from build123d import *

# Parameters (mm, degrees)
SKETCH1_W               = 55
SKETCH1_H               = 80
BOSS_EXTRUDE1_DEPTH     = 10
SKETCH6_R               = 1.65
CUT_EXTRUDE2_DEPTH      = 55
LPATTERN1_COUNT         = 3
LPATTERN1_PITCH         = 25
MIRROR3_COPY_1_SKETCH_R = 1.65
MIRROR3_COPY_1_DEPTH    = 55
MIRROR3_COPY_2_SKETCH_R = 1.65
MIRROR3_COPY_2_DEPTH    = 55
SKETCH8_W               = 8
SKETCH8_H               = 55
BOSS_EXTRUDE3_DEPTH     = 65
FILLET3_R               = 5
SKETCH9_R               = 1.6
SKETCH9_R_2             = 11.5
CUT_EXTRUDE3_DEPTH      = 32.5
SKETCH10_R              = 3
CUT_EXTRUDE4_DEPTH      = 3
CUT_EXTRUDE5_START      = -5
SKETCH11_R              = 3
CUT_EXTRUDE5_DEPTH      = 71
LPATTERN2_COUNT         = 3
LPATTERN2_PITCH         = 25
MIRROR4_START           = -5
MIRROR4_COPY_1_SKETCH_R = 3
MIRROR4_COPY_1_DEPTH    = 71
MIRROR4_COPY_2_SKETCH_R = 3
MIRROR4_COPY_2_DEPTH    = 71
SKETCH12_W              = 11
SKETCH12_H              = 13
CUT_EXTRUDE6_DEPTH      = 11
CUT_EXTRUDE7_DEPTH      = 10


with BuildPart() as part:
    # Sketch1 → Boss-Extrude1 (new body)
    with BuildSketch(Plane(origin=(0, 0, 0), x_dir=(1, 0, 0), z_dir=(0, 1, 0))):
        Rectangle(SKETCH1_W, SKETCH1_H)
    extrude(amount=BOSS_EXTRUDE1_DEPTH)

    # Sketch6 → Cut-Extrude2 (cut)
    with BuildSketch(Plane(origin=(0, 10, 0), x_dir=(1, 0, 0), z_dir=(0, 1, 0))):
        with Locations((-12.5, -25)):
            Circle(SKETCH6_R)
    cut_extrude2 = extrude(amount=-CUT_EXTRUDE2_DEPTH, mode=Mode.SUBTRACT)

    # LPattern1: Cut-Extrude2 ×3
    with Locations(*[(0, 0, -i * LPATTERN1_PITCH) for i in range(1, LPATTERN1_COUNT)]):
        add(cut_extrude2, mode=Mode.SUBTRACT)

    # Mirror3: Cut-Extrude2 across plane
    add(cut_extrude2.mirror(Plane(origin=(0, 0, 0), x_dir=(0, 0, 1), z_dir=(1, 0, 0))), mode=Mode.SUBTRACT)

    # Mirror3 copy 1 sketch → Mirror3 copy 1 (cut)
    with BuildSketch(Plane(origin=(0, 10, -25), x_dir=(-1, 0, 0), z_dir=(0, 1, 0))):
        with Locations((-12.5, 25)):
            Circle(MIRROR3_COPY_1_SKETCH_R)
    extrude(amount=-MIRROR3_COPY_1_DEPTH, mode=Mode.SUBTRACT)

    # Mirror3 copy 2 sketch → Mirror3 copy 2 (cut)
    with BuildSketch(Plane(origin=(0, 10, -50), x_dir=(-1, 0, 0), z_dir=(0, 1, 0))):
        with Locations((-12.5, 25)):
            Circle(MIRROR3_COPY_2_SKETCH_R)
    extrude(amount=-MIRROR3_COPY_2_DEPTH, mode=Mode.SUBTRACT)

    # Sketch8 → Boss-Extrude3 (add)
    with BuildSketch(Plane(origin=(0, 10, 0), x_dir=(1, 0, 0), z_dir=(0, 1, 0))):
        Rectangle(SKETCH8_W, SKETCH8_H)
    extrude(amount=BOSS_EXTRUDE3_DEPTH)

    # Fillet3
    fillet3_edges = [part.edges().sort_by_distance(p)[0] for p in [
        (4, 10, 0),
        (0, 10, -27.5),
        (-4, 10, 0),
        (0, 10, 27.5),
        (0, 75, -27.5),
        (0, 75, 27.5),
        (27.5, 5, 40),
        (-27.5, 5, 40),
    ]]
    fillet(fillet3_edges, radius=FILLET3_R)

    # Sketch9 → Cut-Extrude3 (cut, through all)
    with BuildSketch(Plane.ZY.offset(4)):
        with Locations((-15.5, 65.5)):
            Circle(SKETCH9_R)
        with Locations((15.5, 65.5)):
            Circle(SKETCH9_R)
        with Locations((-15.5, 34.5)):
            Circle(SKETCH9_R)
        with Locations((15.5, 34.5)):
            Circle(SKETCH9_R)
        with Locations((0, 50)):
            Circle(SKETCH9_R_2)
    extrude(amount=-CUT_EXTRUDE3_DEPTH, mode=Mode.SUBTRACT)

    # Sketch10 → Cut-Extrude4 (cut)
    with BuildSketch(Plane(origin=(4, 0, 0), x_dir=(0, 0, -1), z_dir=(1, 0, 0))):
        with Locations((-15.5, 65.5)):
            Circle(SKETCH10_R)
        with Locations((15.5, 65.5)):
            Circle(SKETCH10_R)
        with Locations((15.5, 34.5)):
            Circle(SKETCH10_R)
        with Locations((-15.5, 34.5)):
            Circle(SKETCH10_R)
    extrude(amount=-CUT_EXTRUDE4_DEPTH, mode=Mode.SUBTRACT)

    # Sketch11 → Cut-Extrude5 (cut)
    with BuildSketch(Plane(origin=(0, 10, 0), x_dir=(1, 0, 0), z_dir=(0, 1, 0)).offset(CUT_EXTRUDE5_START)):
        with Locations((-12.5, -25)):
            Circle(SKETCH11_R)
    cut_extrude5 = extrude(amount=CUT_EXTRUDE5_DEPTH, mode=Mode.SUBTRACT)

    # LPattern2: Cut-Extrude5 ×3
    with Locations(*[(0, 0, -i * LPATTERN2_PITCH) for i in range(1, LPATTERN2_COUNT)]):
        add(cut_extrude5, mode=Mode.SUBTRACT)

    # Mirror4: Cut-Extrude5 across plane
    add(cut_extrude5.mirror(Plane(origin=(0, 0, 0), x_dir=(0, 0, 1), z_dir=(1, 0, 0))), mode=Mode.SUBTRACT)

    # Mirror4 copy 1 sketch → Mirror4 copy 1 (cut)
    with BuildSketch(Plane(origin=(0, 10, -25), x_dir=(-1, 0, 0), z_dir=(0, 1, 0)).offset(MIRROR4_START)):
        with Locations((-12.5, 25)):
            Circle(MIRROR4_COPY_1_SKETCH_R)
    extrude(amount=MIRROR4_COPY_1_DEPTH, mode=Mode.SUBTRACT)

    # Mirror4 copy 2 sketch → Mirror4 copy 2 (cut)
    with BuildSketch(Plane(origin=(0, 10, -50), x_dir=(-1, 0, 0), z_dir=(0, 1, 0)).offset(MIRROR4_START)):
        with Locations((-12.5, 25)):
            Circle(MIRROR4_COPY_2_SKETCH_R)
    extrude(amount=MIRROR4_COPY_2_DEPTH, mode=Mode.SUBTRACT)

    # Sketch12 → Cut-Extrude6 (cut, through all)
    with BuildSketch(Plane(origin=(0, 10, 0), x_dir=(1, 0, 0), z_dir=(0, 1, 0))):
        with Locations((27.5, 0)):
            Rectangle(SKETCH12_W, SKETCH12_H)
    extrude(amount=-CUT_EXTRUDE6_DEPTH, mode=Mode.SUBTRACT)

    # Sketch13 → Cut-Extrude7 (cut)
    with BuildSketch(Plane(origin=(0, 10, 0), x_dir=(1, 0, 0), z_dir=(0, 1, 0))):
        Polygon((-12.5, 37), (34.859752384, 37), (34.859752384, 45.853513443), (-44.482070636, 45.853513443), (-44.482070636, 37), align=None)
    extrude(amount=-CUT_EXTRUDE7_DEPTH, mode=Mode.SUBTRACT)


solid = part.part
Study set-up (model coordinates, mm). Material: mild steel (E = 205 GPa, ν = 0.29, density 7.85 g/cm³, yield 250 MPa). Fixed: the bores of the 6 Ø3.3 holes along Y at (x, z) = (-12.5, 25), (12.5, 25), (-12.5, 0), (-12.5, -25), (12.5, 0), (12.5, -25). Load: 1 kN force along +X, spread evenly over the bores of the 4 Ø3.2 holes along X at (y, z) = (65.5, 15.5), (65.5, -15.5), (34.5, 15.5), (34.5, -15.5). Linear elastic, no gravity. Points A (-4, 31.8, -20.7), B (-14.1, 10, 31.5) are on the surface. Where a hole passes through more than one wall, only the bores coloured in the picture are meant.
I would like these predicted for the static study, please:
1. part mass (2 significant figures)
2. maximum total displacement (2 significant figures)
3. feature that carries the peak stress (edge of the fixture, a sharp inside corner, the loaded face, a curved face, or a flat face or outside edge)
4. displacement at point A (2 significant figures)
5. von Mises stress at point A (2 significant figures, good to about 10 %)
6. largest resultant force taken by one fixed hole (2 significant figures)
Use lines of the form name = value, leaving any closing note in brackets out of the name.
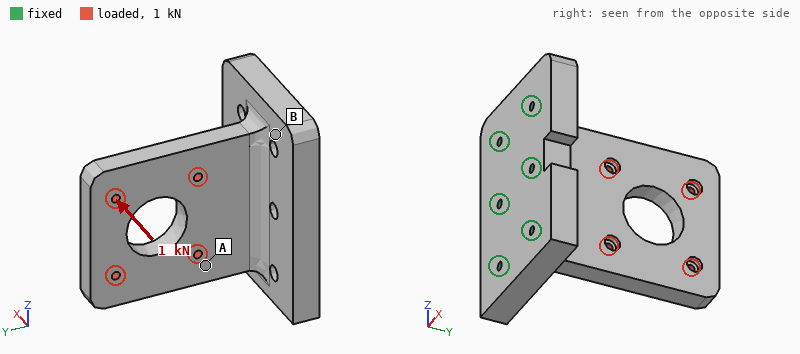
part mass = 520 g
maximum total displacement = 0.10 mm
feature that carries the peak stress = a curved face
displacement at point A = 0.017 mm
von Mises stress at point A = 38 MPa
largest resultant force taken by one fixed hole = 890 N
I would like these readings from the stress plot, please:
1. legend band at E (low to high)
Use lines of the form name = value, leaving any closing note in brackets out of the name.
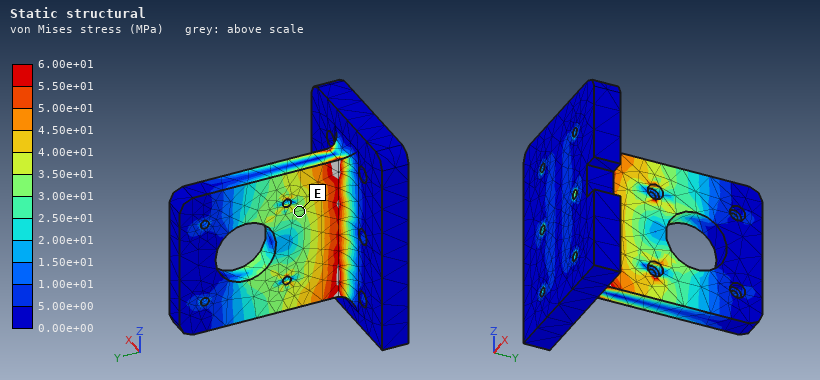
legend band at E = 3.00e+01 to 3.50e+01 MPa
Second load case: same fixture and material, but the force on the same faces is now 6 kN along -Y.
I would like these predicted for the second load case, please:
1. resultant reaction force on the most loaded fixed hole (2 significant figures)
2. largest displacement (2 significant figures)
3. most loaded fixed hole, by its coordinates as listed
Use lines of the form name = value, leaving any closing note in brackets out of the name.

resultant reaction force on the most loaded fixed hole = 1.4 kN
largest displacement = 36 µm
most loaded fixed hole, by its coordinates as listed = (-12.5, 0)
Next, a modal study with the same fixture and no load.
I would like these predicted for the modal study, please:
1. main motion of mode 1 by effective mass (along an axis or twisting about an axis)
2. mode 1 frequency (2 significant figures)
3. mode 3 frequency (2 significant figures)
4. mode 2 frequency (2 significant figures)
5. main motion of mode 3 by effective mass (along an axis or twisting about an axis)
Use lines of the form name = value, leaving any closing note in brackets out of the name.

main motion of mode 1 by effective mass = along X
mode 1 frequency = 1600 Hz
mode 3 frequency = 5900 Hz
mode 2 frequency = 3800 Hz
main motion of mode 3 by effective mass = along Z
